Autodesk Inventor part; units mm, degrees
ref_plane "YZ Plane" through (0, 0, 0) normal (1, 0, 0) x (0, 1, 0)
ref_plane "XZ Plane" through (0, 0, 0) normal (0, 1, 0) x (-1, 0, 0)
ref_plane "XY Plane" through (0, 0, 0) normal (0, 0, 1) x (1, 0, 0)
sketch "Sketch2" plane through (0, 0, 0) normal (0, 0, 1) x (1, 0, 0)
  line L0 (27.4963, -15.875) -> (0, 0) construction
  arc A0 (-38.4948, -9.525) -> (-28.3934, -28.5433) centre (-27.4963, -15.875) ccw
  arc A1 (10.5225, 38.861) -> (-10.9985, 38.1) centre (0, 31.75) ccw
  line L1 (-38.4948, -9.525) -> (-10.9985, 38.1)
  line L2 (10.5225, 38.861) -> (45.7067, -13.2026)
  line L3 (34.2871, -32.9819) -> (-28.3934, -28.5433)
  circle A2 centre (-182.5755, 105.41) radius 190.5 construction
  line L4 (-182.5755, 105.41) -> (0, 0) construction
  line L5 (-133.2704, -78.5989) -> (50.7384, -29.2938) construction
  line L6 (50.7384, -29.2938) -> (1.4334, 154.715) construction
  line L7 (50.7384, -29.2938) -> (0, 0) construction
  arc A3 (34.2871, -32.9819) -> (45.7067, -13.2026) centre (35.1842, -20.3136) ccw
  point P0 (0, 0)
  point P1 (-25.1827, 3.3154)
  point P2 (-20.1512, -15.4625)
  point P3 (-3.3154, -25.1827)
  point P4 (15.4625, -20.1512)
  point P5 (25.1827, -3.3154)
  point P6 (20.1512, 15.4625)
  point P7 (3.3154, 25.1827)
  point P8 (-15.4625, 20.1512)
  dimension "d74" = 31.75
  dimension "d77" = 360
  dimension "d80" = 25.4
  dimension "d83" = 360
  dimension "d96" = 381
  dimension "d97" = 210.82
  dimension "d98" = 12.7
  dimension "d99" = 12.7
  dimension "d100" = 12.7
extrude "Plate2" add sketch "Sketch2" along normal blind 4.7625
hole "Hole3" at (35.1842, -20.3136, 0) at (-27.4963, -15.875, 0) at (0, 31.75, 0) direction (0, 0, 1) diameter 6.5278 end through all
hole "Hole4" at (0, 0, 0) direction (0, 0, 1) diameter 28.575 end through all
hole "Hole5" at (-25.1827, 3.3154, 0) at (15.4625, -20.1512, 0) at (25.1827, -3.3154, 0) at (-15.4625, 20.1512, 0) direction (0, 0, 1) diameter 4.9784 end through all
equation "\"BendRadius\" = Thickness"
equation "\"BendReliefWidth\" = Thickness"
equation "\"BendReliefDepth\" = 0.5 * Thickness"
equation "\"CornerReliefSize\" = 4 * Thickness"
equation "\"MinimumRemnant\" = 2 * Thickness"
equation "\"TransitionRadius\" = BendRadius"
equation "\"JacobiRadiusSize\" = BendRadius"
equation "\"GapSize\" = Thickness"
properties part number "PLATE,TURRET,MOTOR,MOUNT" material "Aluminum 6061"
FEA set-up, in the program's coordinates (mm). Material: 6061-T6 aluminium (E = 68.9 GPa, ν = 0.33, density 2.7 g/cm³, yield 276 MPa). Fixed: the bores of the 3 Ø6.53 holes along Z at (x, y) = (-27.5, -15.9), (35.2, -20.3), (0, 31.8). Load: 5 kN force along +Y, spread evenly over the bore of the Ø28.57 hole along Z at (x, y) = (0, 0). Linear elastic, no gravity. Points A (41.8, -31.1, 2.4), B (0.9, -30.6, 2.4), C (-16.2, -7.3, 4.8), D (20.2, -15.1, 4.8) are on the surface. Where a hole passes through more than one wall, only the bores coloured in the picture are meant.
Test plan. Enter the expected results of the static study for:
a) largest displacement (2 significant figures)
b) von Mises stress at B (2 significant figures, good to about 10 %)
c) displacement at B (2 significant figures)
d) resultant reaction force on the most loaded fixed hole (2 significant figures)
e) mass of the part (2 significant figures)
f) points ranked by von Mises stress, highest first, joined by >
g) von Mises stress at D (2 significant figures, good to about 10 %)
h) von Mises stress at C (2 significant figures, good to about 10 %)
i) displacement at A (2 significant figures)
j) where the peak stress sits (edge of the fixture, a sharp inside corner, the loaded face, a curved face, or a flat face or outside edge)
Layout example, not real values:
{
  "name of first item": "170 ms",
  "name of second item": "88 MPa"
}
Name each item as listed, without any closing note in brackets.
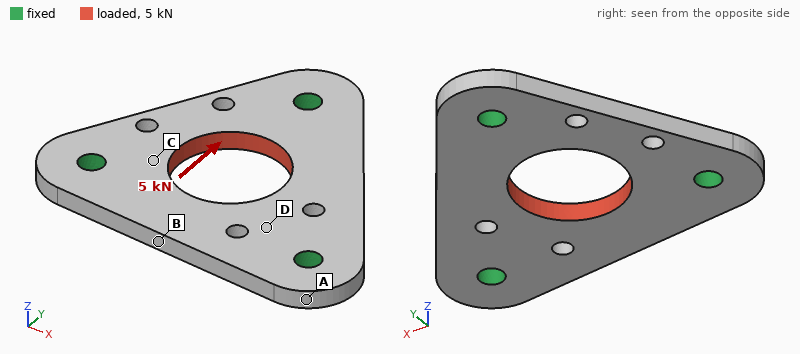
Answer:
{
  "largest displacement": "20 µm",
  "von Mises stress at B": "34 MPa",
  "displacement at B": "18 µm",
  "resultant reaction force on the most loaded fixed hole": "1.9 kN",
  "mass of the part": "45 g",
  "points ranked by von Mises stress, highest first, joined by >": "B > C > D > A",
  "von Mises stress at D": "9.3 MPa",
  "von Mises stress at C": "17 MPa",
  "displacement at A": "3.7 µm",
  "where the peak stress sits": "edge of the fixture"
}
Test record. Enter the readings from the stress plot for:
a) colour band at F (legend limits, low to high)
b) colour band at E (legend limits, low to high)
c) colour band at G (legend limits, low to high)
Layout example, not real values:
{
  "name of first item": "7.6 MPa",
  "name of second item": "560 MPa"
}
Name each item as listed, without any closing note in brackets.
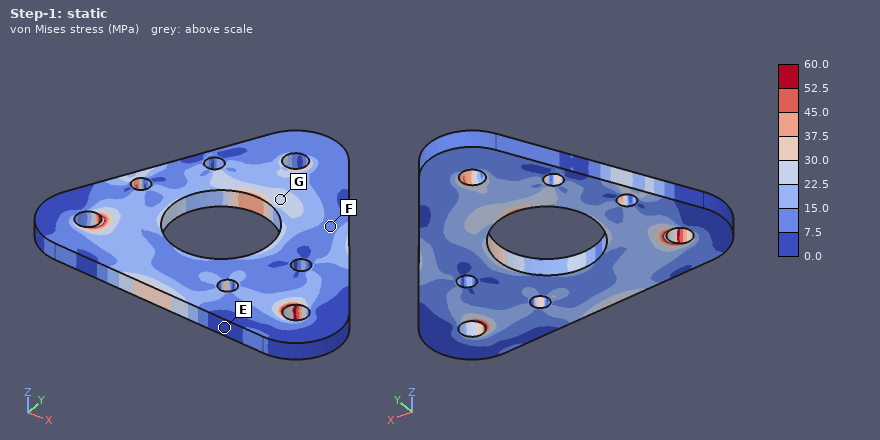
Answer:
{
  "colour band at F": "7.5 to 15.0 MPa",
  "colour band at E": "0.0 to 7.5 MPa",
  "colour band at G": "22.5 to 30.0 MPa"
}
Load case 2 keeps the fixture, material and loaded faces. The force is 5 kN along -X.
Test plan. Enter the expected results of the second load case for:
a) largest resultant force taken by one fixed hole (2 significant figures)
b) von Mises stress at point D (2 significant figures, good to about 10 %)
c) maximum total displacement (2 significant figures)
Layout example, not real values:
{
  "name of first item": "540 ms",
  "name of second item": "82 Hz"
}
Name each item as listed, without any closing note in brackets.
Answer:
{
  "largest resultant force taken by one fixed hole": "1.8 kN",
  "von Mises stress at point D": "14 MPa",
  "maximum total displacement": "16 µm"
}
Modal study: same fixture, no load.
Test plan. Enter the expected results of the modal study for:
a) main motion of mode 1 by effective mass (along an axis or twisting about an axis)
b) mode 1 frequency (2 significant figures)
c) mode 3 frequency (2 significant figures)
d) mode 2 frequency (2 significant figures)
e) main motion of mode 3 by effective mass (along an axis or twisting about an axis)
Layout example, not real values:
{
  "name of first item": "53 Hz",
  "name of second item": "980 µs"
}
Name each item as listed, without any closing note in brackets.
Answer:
{
  "main motion of mode 1 by effective mass": "along Z",
  "mode 1 frequency": "6700 Hz",
  "mode 3 frequency": "9000 Hz",
  "mode 2 frequency": "7100 Hz",
  "main motion of mode 3 by effective mass": "along Z"
}
